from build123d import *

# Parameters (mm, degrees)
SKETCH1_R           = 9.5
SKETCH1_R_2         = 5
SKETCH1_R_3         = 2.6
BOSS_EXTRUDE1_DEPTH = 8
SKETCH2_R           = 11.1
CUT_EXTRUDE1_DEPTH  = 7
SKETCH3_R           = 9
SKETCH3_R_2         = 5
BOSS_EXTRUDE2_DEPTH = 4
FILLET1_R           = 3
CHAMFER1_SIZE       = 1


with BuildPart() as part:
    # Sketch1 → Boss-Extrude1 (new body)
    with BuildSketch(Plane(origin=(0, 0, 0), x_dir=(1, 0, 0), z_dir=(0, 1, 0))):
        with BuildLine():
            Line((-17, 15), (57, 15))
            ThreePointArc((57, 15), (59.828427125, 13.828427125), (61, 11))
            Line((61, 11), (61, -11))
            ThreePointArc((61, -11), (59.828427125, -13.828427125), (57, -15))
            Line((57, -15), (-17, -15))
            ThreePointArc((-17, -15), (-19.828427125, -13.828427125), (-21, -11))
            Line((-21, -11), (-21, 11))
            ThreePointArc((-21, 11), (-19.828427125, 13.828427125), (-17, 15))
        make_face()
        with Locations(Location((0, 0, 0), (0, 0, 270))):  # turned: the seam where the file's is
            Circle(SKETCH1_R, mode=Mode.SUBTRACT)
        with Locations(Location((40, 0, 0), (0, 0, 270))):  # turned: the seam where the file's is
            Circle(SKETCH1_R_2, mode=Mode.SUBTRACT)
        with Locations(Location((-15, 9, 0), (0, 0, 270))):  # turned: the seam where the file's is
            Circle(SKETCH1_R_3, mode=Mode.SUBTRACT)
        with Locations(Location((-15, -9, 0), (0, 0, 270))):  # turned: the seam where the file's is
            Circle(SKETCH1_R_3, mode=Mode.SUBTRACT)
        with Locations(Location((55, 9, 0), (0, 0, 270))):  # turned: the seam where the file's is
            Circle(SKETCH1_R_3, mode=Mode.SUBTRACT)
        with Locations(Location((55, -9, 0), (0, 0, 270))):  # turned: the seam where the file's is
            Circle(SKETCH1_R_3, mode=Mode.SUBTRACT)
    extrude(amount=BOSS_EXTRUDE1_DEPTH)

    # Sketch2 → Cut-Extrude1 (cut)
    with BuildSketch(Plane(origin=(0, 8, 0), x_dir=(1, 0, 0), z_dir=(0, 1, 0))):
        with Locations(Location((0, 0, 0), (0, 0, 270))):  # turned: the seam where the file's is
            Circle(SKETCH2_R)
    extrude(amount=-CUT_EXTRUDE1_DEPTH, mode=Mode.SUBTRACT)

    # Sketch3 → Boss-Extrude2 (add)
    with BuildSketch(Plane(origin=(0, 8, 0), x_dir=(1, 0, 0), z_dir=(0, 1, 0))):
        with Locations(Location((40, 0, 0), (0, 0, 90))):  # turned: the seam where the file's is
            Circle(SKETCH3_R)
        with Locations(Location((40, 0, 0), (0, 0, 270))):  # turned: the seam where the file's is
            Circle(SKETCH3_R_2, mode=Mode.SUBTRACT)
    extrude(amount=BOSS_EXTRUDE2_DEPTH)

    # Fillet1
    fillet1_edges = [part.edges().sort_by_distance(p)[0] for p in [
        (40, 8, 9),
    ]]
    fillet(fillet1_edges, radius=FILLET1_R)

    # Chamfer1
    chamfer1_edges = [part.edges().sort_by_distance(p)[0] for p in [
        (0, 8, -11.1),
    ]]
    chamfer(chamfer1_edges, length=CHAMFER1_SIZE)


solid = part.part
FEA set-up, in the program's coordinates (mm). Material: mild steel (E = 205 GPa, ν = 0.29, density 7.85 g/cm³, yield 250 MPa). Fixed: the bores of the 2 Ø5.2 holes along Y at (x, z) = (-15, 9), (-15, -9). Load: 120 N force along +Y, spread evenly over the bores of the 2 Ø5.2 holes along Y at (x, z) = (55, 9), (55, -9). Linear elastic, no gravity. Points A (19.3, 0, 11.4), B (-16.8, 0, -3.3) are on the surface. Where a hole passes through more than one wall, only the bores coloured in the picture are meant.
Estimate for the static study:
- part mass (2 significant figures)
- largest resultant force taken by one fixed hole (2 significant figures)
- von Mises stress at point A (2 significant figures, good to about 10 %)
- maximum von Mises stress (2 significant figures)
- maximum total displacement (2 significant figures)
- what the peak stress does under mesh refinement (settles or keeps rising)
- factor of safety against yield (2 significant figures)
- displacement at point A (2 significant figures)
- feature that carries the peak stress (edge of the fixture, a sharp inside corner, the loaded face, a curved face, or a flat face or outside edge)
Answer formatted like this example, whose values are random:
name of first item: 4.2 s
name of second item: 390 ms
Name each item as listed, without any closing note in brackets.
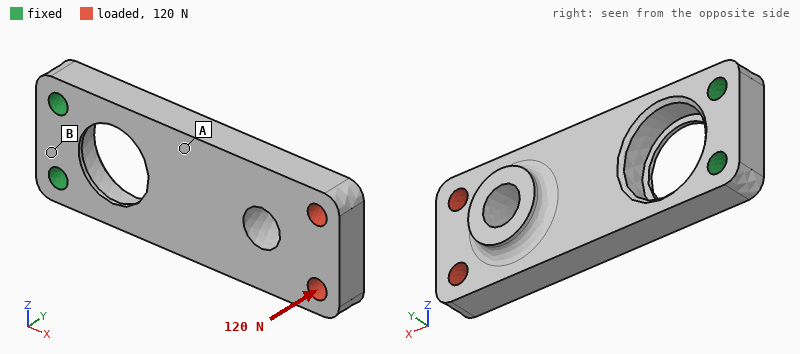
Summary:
part mass: 130 g
largest resultant force taken by one fixed hole: 62 N
von Mises stress at point A: 16 MPa
maximum von Mises stress: 95 MPa
maximum total displacement: 0.13 mm
what the peak stress does under mesh refinement: settles
factor of safety against yield: 2.6
displacement at point A: 0.038 mm
feature that carries the peak stress: a curved face
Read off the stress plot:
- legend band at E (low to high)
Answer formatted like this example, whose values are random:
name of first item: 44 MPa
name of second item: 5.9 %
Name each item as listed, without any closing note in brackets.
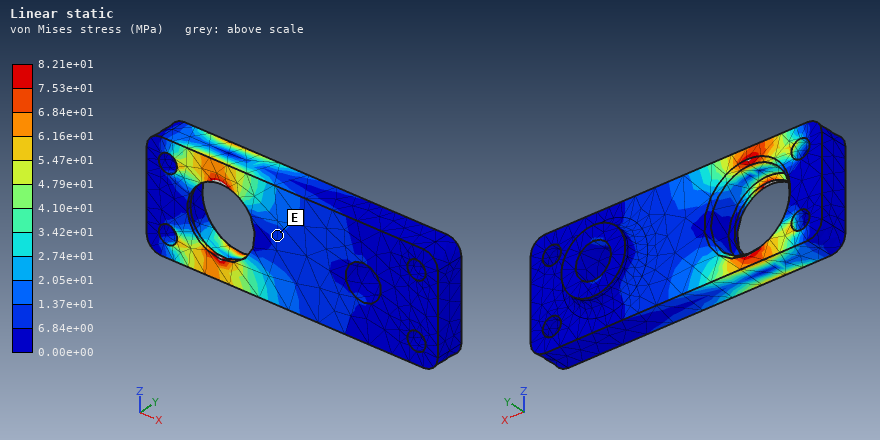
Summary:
legend band at E: 6.84e+00 to 1.37e+01 MPa
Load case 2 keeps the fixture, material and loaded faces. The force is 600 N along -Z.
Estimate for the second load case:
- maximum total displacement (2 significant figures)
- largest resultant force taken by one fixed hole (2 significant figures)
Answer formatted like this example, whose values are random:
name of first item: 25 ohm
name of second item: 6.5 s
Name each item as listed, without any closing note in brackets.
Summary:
maximum total displacement: 43 µm
largest resultant force taken by one fixed hole: 1.6 kN
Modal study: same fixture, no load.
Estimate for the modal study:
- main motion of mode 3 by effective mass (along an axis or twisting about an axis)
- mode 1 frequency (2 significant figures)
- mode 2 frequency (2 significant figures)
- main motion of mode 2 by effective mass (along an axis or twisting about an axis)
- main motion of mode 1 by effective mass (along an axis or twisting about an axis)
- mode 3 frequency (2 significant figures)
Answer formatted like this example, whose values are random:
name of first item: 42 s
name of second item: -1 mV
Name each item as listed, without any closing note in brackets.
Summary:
main motion of mode 3 by effective mass: twisting about X
mode 1 frequency: 780 Hz
mode 2 frequency: 2600 Hz
main motion of mode 2 by effective mass: along Z
main motion of mode 1 by effective mass: along Y
mode 3 frequency: 4200 Hz
